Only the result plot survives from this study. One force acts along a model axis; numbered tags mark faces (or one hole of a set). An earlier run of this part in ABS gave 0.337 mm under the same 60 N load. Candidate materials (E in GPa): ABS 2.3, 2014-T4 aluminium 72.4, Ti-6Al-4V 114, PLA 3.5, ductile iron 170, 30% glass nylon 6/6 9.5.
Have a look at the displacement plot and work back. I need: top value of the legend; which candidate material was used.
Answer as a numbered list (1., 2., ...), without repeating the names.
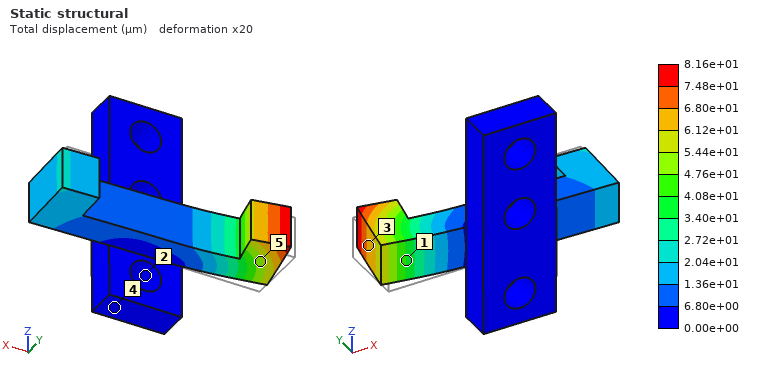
1. 8.16e+01 µm
2. 30% glass nylon 6/6
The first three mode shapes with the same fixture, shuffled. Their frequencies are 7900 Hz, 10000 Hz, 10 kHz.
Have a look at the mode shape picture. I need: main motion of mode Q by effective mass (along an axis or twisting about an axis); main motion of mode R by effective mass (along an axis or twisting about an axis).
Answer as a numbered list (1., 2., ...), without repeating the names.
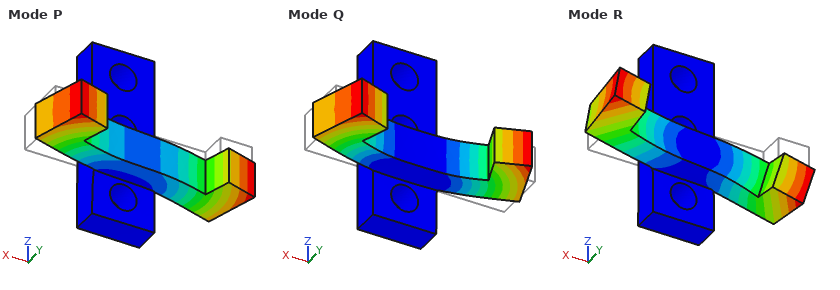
1. along Y
2. twisting about Y
